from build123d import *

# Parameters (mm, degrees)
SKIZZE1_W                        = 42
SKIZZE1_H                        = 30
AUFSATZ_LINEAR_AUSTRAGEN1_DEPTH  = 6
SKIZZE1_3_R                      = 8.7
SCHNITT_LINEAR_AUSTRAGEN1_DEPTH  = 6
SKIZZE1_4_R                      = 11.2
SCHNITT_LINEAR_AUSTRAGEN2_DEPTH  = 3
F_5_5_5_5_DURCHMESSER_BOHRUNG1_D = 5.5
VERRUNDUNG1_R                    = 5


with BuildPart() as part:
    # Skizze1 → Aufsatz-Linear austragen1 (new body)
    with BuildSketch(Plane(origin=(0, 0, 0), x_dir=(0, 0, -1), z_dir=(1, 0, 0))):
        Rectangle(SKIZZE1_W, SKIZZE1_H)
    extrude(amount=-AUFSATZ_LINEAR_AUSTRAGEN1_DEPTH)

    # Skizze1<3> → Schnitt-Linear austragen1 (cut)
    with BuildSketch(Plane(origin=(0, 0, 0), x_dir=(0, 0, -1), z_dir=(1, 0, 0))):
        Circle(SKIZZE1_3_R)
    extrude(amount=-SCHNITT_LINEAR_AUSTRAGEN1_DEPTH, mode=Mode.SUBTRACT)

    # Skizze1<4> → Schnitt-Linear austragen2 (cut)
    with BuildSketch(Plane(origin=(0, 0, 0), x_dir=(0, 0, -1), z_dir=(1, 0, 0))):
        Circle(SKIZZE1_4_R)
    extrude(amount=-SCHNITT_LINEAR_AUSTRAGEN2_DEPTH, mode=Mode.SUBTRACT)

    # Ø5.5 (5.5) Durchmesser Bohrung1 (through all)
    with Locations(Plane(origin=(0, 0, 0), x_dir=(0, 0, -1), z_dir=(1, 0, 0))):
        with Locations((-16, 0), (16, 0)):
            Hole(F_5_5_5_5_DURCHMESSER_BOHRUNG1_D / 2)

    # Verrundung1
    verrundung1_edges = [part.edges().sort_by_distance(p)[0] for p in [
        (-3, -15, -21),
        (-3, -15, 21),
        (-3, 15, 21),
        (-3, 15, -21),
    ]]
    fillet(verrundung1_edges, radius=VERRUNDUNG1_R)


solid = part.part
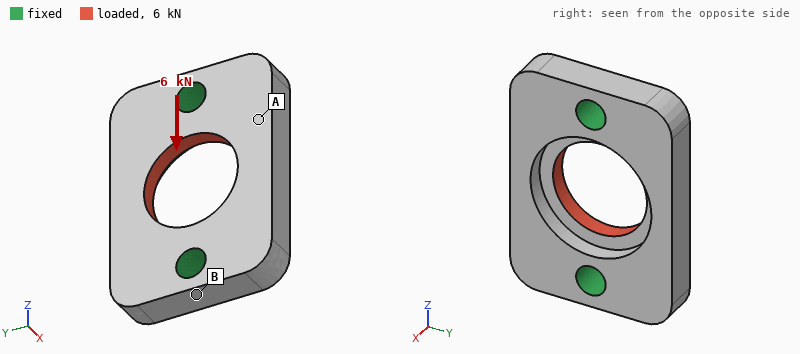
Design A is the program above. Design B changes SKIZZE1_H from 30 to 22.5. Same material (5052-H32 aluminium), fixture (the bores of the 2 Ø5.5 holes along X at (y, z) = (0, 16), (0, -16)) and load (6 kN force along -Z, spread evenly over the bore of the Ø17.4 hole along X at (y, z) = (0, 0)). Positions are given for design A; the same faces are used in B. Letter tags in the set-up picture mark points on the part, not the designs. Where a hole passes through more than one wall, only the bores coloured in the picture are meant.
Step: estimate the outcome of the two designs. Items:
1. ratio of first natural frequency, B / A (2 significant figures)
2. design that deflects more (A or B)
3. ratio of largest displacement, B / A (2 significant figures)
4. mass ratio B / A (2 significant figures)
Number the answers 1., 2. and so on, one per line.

1. 1.6
2. B
3. 1.2
4. 0.64
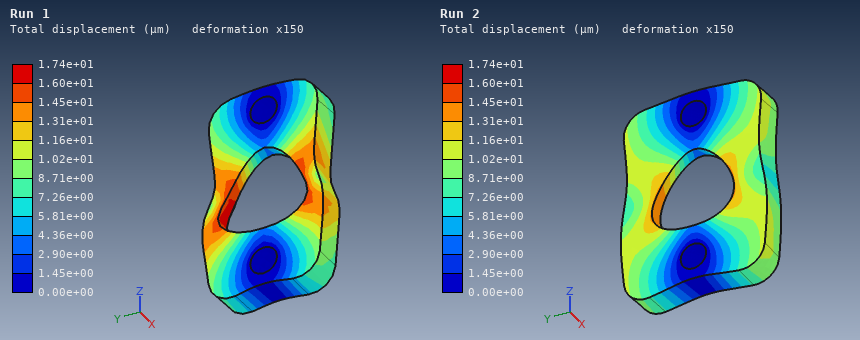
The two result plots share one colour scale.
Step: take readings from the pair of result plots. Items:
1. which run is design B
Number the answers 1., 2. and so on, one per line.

1. Run 1
